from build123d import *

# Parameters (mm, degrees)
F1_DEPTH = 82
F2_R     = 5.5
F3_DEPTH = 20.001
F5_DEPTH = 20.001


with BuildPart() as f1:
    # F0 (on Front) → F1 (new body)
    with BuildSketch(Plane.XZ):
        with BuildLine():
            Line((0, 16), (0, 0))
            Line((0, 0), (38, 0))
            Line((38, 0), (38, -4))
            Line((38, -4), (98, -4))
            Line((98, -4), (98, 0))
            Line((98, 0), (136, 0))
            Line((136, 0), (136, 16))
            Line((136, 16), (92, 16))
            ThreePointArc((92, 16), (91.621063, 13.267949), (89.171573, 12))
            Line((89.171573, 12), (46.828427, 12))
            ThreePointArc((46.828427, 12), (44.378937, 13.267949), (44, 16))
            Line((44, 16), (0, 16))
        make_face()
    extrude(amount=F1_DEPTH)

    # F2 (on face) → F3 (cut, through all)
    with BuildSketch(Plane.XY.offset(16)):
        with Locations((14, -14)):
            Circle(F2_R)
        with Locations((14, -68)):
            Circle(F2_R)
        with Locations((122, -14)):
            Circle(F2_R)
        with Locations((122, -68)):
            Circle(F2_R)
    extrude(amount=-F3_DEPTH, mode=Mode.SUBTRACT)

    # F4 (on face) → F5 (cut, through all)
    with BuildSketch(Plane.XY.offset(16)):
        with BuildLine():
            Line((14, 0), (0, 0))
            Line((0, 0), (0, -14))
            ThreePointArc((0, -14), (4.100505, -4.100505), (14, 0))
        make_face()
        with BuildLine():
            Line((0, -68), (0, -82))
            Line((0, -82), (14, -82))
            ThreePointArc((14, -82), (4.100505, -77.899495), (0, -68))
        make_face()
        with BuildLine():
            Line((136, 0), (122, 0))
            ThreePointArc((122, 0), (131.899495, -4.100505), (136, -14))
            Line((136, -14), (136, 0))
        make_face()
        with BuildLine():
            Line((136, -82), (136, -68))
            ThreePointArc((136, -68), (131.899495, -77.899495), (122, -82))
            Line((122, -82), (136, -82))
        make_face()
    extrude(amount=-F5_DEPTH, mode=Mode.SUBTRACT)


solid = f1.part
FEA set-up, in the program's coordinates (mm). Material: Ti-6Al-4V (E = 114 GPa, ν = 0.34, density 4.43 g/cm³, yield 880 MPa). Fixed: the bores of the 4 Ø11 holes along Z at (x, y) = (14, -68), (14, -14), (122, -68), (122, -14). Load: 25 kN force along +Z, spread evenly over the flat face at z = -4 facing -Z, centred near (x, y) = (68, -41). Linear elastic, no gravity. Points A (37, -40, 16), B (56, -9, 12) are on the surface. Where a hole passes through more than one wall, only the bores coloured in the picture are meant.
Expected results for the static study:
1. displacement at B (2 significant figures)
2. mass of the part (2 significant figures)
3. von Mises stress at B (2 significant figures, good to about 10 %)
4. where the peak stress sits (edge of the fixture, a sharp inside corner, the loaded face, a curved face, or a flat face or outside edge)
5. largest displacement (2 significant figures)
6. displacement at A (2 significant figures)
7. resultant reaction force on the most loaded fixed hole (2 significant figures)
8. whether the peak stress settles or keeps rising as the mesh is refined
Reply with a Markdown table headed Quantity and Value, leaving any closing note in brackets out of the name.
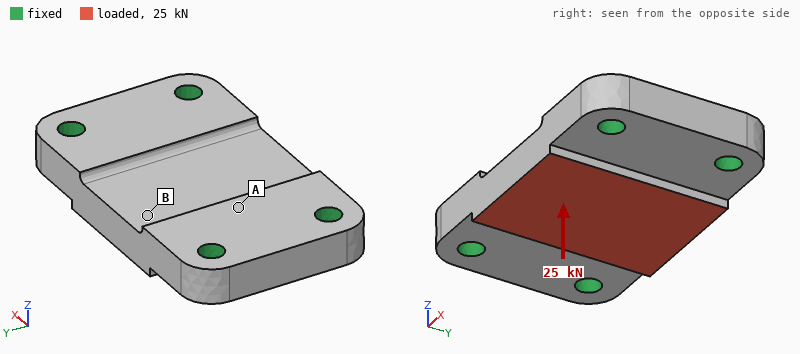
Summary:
| Quantity | Value |
|---|---|
| displacement at B | 40 µm |
| mass of the part | 770 g |
| von Mises stress at B | 32 MPa |
| where the peak stress sits | edge of the fixture |
| largest displacement | 46 µm |
| displacement at A | 25 µm |
| resultant reaction force on the most loaded fixed hole | 8.1 kN |
| whether the peak stress settles or keeps rising as the mesh is refined | keeps rising |
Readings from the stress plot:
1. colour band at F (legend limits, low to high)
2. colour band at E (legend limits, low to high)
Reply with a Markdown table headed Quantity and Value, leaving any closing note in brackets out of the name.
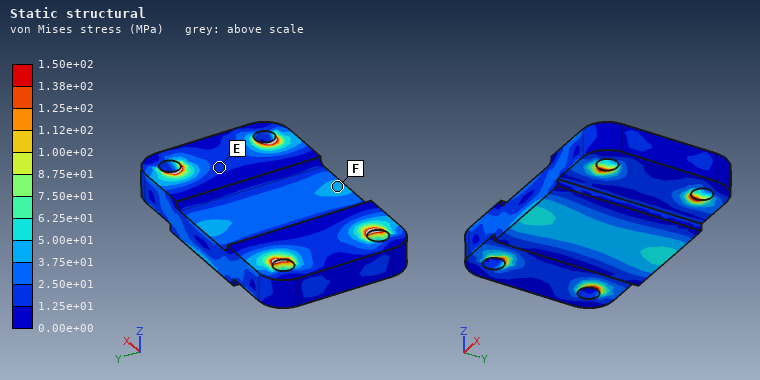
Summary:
| Quantity | Value |
|---|---|
| colour band at F | 3.75e+01 to 5.00e+01 MPa |
| colour band at E | 1.25e+01 to 2.50e+01 MPa |
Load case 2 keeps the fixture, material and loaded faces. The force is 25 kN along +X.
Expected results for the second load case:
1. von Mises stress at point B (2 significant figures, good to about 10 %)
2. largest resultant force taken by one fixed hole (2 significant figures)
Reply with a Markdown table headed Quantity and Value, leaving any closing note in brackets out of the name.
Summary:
| Quantity | Value |
|---|---|
| von Mises stress at point B | 4.1 MPa |
| largest resultant force taken by one fixed hole | 6.6 kN |
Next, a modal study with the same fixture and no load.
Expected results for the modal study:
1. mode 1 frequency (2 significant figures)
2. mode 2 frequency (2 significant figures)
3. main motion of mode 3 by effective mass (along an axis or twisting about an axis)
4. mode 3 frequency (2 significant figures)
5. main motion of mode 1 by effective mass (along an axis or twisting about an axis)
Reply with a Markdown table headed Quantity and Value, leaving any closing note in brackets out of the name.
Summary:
| Quantity | Value |
|---|---|
| mode 1 frequency | 6500 Hz |
| mode 2 frequency | 8400 Hz |
| main motion of mode 3 by effective mass | along Y |
| mode 3 frequency | 12 kHz |
| main motion of mode 1 by effective mass | along Z |
